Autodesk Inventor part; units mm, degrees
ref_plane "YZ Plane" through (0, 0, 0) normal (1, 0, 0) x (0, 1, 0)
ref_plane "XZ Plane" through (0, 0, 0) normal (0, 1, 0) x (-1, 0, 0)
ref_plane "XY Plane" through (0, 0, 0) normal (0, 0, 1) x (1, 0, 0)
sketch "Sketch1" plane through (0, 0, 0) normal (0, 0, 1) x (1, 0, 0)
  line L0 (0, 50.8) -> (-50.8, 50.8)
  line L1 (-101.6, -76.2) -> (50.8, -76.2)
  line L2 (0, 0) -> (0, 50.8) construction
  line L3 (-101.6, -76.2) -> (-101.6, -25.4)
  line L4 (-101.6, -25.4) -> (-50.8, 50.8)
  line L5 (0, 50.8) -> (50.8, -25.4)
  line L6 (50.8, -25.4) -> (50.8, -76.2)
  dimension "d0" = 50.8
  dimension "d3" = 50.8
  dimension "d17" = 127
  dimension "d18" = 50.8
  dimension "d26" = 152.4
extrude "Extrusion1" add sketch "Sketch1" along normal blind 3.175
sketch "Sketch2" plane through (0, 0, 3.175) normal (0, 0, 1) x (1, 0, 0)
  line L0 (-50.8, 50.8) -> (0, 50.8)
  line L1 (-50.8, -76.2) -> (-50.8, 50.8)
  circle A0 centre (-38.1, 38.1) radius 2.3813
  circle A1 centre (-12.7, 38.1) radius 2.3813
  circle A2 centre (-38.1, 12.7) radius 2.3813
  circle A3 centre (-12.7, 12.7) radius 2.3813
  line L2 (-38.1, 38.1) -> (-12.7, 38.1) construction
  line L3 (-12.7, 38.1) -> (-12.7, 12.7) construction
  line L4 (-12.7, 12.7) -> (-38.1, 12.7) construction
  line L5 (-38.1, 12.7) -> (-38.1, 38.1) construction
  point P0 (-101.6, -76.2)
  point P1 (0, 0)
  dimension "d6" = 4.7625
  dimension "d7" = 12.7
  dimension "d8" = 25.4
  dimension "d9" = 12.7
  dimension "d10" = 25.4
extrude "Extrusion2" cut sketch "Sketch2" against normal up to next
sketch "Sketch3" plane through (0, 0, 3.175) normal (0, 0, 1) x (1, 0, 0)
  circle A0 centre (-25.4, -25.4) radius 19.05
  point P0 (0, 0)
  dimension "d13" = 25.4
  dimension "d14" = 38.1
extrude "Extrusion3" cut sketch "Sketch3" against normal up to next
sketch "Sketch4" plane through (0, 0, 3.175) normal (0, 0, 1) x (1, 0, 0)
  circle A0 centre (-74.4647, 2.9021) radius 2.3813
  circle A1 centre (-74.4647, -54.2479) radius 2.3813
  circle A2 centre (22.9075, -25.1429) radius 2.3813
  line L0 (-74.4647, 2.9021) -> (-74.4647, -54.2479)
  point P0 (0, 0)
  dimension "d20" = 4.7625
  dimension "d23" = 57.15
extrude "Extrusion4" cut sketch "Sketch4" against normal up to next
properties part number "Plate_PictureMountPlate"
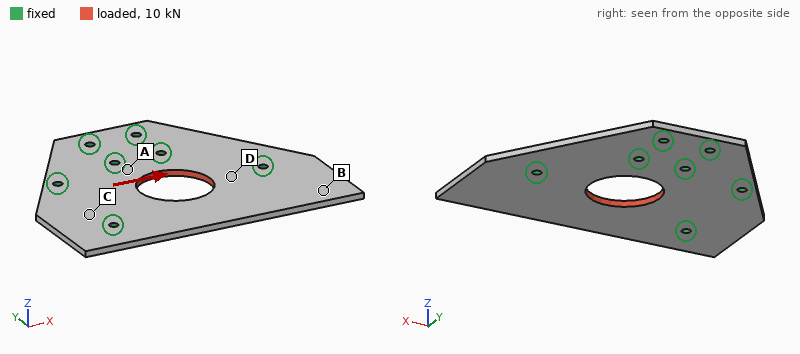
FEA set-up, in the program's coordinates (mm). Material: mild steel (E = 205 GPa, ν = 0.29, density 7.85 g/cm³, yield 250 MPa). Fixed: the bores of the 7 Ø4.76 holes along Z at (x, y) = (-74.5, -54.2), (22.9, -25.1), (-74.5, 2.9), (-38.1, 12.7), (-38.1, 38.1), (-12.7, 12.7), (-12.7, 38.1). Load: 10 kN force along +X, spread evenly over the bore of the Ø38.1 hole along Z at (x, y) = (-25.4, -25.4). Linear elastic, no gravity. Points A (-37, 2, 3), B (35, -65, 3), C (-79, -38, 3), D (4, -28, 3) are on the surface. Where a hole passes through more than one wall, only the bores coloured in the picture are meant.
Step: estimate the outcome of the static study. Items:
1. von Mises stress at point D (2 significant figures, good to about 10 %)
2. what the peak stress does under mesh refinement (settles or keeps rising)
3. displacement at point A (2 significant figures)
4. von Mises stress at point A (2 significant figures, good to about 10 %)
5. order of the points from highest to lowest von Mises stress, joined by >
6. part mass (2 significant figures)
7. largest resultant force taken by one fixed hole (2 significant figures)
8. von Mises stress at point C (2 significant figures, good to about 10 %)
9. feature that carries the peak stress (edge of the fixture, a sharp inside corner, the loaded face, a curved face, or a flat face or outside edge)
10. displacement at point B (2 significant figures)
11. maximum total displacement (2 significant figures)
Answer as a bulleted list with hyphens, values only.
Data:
- 35 MPa
- keeps rising
- 2.0 µm
- 23 MPa
- D > A > C > B
- 350 g
- 3.0 kN
- 14 MPa
- edge of the fixture
- 5.6 µm
- 8.1 µm
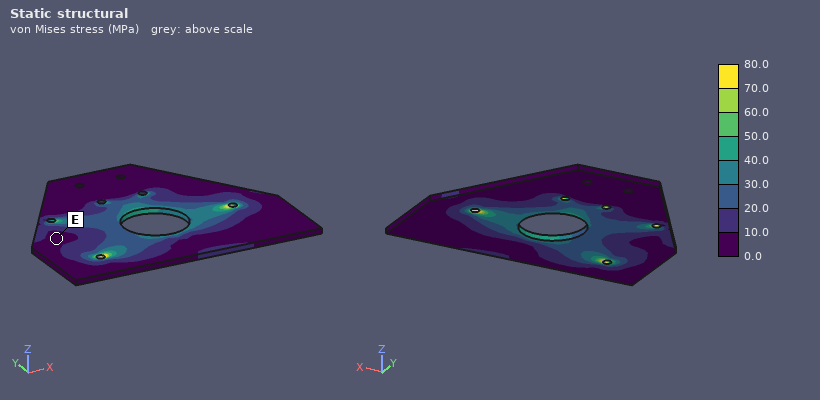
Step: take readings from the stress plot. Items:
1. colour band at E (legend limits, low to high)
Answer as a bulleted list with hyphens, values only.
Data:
- 0.0 to 10.0 MPa
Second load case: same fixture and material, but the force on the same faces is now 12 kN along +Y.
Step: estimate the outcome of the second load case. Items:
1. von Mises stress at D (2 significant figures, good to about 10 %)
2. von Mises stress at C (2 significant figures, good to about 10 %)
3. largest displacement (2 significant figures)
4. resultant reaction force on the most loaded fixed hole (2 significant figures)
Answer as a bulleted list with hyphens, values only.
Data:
- 26 MPa
- 10 MPa
- 15 µm
- 2.8 kN
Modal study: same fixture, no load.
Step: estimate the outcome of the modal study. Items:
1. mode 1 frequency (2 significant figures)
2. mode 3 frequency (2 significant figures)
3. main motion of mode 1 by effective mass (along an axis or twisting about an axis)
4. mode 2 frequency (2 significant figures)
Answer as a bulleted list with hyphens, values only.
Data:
- 960 Hz
- 2900 Hz
- along Z
- 1500 Hz
